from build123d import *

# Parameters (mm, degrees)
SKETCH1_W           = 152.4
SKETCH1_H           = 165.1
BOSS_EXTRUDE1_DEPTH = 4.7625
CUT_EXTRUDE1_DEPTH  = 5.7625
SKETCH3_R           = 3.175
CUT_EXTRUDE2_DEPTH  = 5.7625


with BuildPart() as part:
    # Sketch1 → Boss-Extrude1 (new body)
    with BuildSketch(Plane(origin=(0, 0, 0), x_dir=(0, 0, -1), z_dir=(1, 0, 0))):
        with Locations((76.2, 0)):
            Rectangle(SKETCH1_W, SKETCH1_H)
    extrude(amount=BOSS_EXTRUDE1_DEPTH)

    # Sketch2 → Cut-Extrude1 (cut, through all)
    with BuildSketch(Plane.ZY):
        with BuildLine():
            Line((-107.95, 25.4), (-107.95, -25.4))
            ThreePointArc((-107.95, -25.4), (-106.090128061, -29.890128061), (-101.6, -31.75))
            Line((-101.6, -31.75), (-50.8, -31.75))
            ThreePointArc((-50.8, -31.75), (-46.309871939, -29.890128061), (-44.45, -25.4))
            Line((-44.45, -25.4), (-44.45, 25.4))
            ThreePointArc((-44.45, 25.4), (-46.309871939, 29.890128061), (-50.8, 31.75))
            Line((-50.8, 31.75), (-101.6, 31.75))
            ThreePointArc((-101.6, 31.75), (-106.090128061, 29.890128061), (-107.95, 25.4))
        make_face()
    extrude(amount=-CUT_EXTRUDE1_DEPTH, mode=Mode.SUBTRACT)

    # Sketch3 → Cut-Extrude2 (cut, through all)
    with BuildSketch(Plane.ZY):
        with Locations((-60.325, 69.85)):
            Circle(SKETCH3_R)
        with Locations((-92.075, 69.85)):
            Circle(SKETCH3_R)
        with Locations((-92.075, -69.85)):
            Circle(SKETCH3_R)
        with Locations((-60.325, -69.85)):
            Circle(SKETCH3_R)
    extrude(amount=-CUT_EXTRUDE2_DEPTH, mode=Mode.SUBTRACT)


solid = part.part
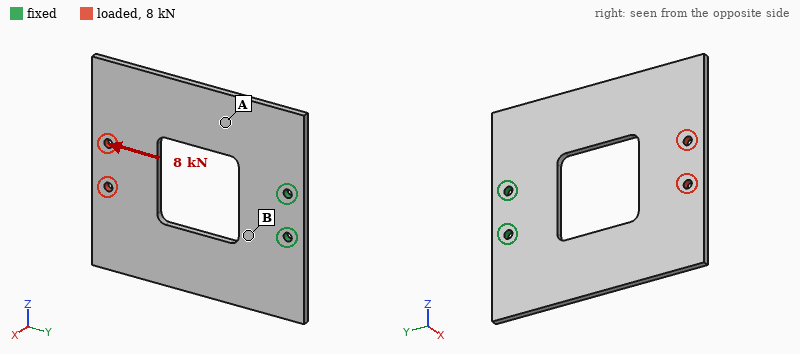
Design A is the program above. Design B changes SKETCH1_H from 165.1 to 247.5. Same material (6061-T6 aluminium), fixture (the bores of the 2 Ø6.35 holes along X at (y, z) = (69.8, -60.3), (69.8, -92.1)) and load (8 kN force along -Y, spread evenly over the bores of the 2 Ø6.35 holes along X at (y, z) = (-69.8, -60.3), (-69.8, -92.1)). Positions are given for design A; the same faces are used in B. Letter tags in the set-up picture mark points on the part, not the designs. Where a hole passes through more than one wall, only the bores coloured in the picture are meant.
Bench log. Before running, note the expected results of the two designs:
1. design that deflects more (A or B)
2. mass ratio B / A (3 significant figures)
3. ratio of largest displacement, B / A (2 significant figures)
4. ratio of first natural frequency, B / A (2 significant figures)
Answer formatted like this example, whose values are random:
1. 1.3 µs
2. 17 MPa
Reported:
1. A
2. 1.60
3. 0.63
4. 0.63
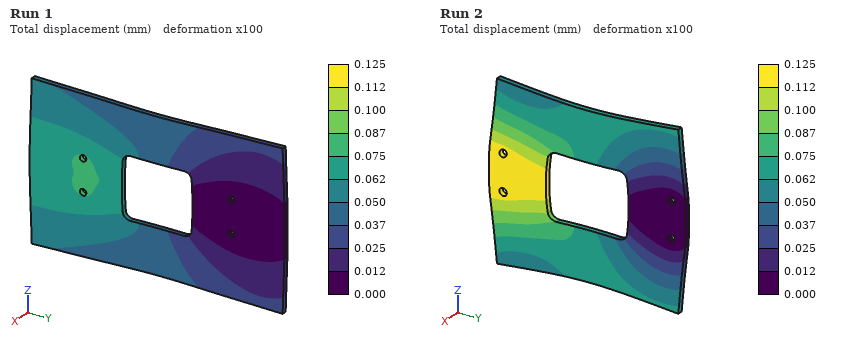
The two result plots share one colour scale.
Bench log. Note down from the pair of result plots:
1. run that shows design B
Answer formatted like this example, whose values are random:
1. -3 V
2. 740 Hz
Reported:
1. Run 1
